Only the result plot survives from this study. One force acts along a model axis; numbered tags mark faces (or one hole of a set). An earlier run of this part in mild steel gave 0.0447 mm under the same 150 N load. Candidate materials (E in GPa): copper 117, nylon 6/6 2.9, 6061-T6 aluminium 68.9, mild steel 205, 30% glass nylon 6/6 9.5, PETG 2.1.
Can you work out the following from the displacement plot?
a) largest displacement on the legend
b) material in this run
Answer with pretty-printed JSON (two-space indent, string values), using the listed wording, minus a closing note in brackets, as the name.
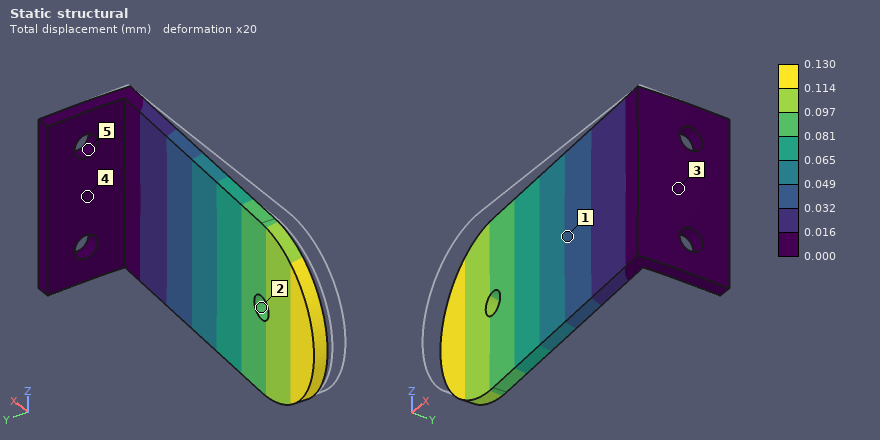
{
  "largest displacement on the legend": "0.130 mm",
  "material in this run": "6061-T6 aluminium"
}
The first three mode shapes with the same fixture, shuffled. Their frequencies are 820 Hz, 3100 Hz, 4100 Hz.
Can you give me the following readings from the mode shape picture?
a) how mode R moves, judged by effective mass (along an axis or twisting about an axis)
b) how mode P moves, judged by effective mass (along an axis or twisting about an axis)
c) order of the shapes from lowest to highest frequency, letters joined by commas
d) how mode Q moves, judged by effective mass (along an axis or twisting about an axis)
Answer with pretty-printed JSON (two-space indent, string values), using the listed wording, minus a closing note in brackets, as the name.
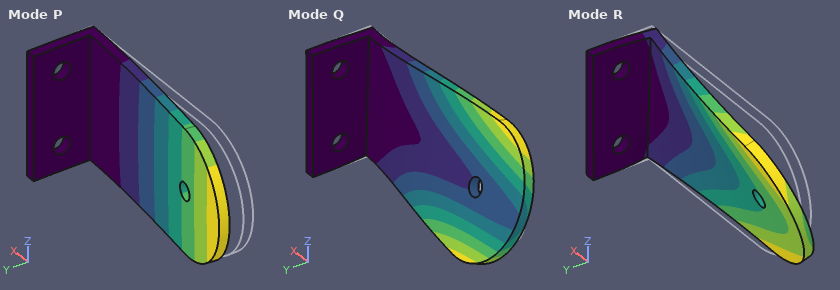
{
  "how mode R moves, judged by effective mass": "along Z",
  "how mode P moves, judged by effective mass": "along Y",
  "order of the shapes from lowest to highest frequency, letters joined by commas": "P, R, Q",
  "how mode Q moves, judged by effective mass": "along Z"
}
